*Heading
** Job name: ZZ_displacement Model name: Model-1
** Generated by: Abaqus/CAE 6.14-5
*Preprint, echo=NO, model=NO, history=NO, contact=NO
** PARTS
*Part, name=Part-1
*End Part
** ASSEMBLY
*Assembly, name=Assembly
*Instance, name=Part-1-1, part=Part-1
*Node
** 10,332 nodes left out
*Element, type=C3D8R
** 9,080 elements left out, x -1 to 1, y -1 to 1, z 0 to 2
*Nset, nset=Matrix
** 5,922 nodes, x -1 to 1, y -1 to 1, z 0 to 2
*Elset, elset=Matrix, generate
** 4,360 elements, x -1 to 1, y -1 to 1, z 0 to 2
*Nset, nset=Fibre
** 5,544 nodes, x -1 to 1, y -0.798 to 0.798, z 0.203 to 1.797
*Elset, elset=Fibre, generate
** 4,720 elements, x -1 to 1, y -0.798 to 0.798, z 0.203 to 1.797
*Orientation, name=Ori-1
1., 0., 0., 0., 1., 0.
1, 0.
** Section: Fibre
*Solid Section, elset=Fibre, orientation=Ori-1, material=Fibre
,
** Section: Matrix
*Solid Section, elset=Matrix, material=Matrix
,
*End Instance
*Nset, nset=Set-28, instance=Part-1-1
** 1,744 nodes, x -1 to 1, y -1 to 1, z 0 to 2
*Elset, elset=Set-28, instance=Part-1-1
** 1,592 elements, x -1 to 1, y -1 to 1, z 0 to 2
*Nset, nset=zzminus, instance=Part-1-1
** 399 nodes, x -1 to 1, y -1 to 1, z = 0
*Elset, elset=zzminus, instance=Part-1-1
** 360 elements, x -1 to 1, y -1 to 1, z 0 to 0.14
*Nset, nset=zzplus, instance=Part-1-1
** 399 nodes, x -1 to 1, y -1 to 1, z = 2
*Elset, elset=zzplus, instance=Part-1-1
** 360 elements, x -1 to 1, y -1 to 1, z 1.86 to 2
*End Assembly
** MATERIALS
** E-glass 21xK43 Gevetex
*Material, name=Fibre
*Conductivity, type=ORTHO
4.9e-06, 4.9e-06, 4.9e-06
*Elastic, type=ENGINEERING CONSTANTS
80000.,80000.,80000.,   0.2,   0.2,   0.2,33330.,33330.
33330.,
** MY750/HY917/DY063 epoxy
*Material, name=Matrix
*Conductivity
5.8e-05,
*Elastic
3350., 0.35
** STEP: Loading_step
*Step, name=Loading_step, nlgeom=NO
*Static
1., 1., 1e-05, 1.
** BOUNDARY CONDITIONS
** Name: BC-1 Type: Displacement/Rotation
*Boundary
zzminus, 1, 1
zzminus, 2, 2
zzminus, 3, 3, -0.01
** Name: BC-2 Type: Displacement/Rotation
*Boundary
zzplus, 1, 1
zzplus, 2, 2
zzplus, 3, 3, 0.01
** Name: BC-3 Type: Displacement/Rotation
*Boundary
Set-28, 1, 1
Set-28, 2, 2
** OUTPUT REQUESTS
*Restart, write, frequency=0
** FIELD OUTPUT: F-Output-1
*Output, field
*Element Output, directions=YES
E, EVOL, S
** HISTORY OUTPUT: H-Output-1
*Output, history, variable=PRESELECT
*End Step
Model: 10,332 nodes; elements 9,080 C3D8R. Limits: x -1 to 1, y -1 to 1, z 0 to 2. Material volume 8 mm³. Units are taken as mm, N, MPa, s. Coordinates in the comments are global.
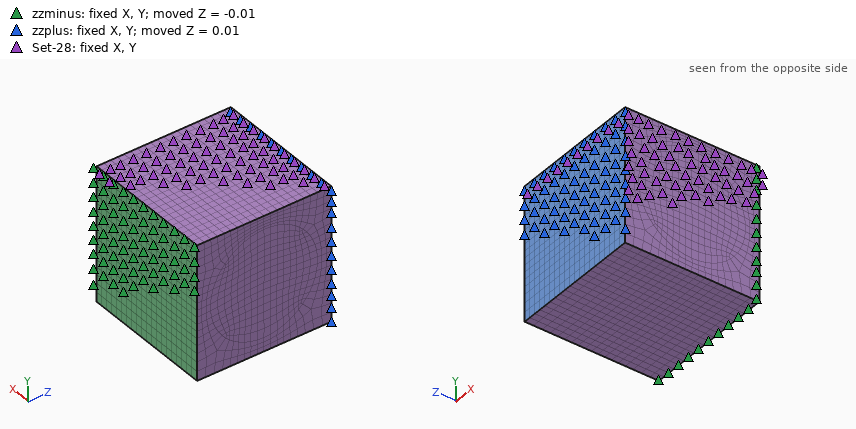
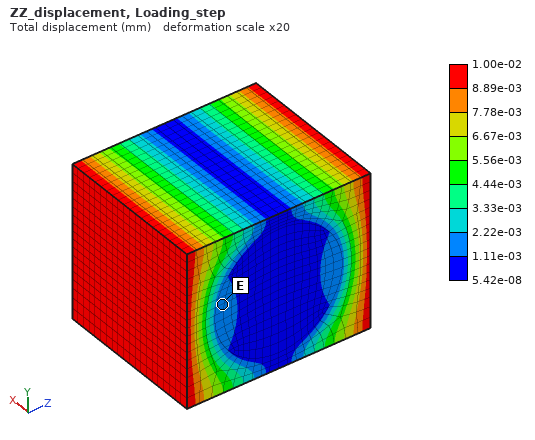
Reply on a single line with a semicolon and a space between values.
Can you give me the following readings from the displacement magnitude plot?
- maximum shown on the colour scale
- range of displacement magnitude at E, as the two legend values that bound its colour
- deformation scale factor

1.00e-02 mm; 1.11e-03 to 2.22e-03 mm; 20
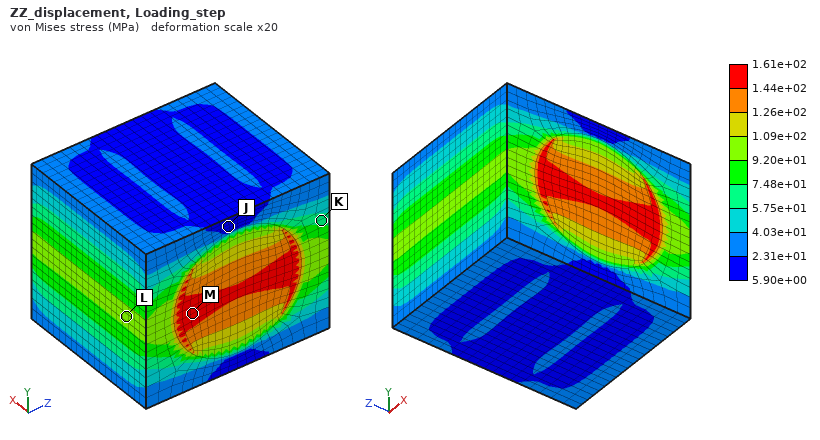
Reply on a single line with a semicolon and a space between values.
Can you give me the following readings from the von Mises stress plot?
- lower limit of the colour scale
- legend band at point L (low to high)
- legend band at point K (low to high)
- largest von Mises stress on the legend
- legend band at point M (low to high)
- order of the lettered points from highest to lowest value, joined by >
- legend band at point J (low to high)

5.90e+00 MPa; 9.20e+01 to 1.09e+02 MPa; 5.75e+01 to 7.48e+01 MPa; 1.61e+02 MPa; 1.44e+02 to 1.61e+02 MPa; M > L > K > J; 5.90e+00 to 2.31e+01 MPa
